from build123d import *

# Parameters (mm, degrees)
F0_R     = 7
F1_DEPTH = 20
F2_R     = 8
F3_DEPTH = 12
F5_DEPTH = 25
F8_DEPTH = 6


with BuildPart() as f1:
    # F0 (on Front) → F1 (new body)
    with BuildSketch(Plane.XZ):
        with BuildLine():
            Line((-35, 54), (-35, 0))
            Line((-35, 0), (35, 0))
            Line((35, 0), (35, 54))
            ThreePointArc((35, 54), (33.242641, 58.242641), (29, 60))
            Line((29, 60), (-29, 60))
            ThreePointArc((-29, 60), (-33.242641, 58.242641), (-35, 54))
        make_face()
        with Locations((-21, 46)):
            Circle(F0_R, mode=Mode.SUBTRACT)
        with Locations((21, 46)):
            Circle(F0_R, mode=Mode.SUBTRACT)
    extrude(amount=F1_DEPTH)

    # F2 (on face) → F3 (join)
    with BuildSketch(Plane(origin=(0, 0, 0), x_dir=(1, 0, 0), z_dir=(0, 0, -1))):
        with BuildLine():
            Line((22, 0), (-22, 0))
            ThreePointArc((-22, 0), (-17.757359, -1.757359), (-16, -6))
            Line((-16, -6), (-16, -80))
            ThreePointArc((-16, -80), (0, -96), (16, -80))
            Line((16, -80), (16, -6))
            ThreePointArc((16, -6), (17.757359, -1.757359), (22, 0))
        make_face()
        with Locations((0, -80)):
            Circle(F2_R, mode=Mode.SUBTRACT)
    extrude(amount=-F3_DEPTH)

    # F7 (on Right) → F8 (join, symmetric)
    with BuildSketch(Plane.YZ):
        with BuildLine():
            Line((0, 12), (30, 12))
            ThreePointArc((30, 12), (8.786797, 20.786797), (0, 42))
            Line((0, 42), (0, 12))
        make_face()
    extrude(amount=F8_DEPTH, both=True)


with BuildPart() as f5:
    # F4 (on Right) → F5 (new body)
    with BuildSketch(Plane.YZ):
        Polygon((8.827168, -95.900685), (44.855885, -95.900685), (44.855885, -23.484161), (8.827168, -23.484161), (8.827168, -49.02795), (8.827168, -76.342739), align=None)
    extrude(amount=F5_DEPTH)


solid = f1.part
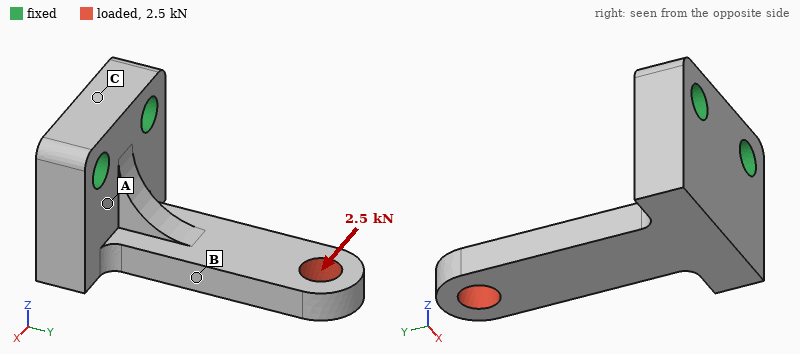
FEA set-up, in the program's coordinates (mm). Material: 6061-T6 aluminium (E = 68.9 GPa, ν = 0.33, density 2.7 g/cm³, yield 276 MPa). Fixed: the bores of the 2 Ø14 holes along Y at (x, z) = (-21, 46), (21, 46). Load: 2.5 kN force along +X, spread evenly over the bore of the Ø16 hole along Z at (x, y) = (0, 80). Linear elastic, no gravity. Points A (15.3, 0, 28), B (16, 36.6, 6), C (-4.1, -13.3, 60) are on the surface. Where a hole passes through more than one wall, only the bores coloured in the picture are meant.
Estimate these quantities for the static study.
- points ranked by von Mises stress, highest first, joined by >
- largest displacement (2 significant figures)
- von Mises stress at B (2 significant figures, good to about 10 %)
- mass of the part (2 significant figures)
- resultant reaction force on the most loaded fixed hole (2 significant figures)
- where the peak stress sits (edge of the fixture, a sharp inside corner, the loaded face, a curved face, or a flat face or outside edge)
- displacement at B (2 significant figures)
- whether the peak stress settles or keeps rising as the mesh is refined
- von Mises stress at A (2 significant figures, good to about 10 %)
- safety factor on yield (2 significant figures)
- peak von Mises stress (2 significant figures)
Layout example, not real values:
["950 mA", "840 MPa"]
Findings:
["B > A > C", "0.44 mm", "53 MPa", "310 g", "4.9 kN", "a curved face", "0.15 mm", "settles", "29 MPa", "1.6", "170 MPa"]
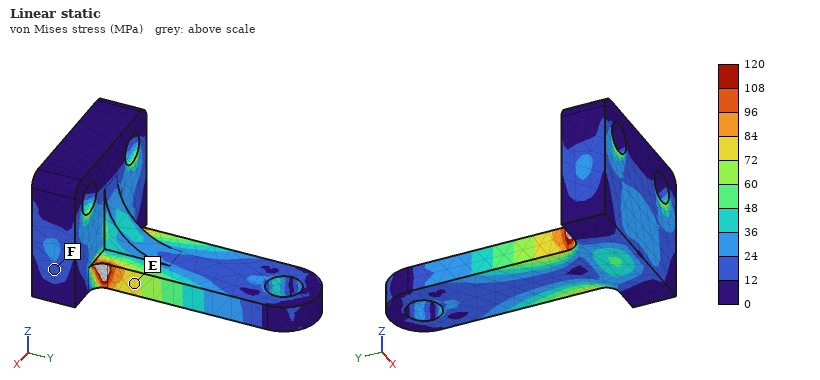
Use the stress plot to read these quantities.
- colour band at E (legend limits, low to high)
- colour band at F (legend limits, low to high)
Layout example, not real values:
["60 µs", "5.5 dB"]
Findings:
["72 to 84 MPa", "12 to 24 MPa"]
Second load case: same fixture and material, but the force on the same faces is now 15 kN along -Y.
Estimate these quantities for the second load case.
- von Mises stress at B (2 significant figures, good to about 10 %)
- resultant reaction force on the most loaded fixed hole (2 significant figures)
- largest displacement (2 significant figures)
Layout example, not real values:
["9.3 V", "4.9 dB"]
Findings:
["38 MPa", "7.5 kN", "0.44 mm"]
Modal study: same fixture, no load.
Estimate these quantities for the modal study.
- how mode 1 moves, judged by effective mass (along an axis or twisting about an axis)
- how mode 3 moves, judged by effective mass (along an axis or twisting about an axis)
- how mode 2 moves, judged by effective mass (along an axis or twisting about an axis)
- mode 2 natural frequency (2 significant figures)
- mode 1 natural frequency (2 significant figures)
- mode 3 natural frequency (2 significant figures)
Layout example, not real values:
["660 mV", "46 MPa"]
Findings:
["along Z", "along Y", "along X", "2300 Hz", "1300 Hz", "4700 Hz"]
